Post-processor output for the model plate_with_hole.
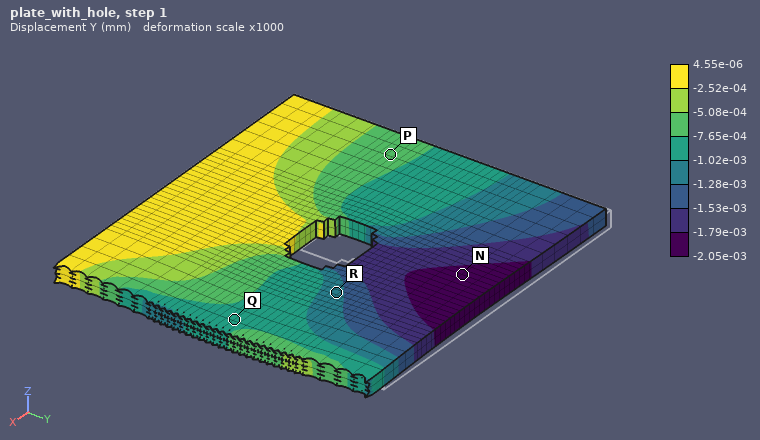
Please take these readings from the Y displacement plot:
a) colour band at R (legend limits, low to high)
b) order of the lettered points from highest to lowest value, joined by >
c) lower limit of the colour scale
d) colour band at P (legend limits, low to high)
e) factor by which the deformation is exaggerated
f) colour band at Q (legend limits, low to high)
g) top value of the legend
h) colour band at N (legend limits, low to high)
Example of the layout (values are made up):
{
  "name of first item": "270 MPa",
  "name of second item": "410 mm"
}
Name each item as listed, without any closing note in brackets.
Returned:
{
  "colour band at R": "-1.28e-03 to -1.02e-03 mm",
  "order of the lettered points from highest to lowest value, joined by >": "P > Q > R > N",
  "lower limit of the colour scale": "-2.05e-03 mm",
  "colour band at P": "-7.65e-04 to -5.08e-04 mm",
  "factor by which the deformation is exaggerated": "1000",
  "colour band at Q": "-1.02e-03 to -7.65e-04 mm",
  "top value of the legend": "4.55e-06 mm",
  "colour band at N": "-2.05e-03 to -1.79e-03 mm"
}
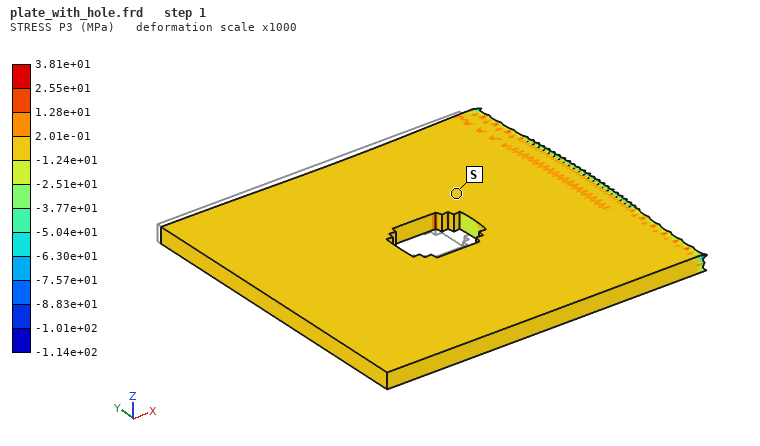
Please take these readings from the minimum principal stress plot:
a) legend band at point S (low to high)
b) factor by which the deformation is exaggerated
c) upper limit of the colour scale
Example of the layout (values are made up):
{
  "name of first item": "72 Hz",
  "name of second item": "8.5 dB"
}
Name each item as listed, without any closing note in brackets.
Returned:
{
  "legend band at point S": "-1.24e+01 to 2.01e-01 MPa",
  "factor by which the deformation is exaggerated": "1000",
  "upper limit of the colour scale": "3.81e+01 MPa"
}
